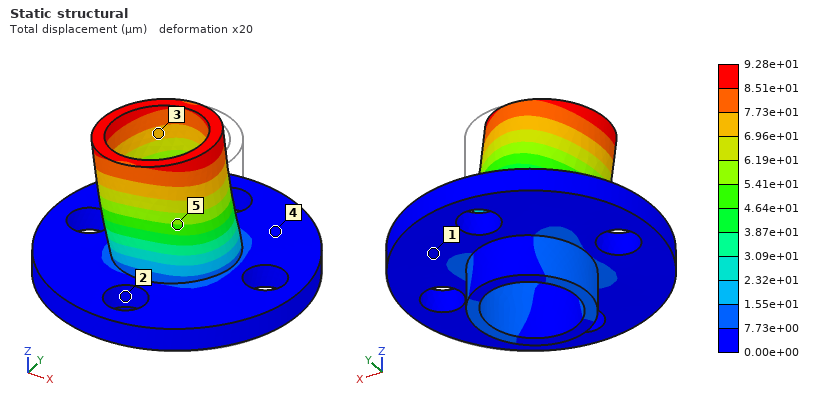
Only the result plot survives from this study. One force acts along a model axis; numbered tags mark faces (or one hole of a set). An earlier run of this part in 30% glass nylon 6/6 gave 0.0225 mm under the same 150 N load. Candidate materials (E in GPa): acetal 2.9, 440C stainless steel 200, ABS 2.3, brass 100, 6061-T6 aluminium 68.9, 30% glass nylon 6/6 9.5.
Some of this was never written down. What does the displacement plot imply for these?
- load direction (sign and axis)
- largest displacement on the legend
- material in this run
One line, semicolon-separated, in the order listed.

-X; 9.28e+01 µm; ABS
